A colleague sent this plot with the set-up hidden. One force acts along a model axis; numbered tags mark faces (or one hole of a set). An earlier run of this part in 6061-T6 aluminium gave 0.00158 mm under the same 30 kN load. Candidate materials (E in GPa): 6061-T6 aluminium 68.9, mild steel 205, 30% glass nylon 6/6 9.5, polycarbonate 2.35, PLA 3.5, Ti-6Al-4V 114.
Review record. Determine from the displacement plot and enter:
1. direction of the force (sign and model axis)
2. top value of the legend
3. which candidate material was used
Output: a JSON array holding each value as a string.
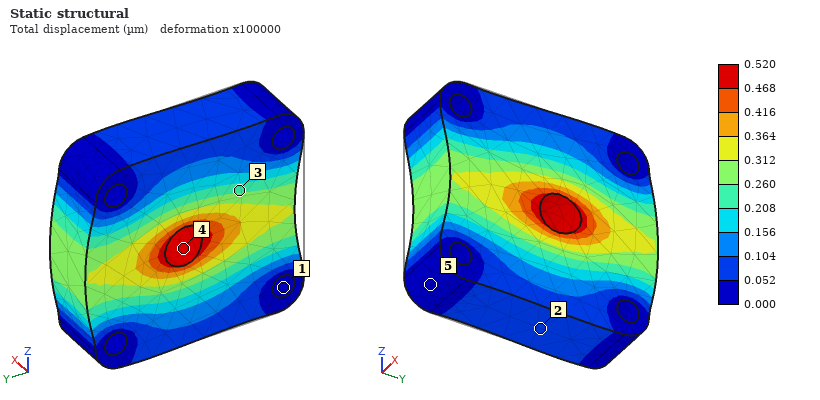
["+Y", "0.520 µm", "mild steel"]
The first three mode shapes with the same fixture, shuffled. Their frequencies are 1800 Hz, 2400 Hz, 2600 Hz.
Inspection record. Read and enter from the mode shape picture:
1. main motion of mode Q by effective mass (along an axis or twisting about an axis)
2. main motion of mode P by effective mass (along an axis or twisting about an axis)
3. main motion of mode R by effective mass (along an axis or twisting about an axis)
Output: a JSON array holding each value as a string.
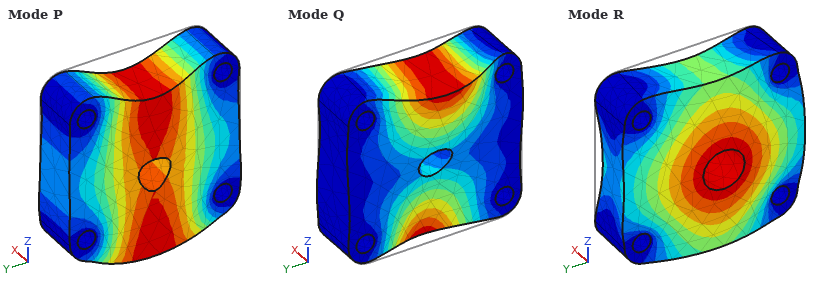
["twisting about Y", "along Z", "along X"]
